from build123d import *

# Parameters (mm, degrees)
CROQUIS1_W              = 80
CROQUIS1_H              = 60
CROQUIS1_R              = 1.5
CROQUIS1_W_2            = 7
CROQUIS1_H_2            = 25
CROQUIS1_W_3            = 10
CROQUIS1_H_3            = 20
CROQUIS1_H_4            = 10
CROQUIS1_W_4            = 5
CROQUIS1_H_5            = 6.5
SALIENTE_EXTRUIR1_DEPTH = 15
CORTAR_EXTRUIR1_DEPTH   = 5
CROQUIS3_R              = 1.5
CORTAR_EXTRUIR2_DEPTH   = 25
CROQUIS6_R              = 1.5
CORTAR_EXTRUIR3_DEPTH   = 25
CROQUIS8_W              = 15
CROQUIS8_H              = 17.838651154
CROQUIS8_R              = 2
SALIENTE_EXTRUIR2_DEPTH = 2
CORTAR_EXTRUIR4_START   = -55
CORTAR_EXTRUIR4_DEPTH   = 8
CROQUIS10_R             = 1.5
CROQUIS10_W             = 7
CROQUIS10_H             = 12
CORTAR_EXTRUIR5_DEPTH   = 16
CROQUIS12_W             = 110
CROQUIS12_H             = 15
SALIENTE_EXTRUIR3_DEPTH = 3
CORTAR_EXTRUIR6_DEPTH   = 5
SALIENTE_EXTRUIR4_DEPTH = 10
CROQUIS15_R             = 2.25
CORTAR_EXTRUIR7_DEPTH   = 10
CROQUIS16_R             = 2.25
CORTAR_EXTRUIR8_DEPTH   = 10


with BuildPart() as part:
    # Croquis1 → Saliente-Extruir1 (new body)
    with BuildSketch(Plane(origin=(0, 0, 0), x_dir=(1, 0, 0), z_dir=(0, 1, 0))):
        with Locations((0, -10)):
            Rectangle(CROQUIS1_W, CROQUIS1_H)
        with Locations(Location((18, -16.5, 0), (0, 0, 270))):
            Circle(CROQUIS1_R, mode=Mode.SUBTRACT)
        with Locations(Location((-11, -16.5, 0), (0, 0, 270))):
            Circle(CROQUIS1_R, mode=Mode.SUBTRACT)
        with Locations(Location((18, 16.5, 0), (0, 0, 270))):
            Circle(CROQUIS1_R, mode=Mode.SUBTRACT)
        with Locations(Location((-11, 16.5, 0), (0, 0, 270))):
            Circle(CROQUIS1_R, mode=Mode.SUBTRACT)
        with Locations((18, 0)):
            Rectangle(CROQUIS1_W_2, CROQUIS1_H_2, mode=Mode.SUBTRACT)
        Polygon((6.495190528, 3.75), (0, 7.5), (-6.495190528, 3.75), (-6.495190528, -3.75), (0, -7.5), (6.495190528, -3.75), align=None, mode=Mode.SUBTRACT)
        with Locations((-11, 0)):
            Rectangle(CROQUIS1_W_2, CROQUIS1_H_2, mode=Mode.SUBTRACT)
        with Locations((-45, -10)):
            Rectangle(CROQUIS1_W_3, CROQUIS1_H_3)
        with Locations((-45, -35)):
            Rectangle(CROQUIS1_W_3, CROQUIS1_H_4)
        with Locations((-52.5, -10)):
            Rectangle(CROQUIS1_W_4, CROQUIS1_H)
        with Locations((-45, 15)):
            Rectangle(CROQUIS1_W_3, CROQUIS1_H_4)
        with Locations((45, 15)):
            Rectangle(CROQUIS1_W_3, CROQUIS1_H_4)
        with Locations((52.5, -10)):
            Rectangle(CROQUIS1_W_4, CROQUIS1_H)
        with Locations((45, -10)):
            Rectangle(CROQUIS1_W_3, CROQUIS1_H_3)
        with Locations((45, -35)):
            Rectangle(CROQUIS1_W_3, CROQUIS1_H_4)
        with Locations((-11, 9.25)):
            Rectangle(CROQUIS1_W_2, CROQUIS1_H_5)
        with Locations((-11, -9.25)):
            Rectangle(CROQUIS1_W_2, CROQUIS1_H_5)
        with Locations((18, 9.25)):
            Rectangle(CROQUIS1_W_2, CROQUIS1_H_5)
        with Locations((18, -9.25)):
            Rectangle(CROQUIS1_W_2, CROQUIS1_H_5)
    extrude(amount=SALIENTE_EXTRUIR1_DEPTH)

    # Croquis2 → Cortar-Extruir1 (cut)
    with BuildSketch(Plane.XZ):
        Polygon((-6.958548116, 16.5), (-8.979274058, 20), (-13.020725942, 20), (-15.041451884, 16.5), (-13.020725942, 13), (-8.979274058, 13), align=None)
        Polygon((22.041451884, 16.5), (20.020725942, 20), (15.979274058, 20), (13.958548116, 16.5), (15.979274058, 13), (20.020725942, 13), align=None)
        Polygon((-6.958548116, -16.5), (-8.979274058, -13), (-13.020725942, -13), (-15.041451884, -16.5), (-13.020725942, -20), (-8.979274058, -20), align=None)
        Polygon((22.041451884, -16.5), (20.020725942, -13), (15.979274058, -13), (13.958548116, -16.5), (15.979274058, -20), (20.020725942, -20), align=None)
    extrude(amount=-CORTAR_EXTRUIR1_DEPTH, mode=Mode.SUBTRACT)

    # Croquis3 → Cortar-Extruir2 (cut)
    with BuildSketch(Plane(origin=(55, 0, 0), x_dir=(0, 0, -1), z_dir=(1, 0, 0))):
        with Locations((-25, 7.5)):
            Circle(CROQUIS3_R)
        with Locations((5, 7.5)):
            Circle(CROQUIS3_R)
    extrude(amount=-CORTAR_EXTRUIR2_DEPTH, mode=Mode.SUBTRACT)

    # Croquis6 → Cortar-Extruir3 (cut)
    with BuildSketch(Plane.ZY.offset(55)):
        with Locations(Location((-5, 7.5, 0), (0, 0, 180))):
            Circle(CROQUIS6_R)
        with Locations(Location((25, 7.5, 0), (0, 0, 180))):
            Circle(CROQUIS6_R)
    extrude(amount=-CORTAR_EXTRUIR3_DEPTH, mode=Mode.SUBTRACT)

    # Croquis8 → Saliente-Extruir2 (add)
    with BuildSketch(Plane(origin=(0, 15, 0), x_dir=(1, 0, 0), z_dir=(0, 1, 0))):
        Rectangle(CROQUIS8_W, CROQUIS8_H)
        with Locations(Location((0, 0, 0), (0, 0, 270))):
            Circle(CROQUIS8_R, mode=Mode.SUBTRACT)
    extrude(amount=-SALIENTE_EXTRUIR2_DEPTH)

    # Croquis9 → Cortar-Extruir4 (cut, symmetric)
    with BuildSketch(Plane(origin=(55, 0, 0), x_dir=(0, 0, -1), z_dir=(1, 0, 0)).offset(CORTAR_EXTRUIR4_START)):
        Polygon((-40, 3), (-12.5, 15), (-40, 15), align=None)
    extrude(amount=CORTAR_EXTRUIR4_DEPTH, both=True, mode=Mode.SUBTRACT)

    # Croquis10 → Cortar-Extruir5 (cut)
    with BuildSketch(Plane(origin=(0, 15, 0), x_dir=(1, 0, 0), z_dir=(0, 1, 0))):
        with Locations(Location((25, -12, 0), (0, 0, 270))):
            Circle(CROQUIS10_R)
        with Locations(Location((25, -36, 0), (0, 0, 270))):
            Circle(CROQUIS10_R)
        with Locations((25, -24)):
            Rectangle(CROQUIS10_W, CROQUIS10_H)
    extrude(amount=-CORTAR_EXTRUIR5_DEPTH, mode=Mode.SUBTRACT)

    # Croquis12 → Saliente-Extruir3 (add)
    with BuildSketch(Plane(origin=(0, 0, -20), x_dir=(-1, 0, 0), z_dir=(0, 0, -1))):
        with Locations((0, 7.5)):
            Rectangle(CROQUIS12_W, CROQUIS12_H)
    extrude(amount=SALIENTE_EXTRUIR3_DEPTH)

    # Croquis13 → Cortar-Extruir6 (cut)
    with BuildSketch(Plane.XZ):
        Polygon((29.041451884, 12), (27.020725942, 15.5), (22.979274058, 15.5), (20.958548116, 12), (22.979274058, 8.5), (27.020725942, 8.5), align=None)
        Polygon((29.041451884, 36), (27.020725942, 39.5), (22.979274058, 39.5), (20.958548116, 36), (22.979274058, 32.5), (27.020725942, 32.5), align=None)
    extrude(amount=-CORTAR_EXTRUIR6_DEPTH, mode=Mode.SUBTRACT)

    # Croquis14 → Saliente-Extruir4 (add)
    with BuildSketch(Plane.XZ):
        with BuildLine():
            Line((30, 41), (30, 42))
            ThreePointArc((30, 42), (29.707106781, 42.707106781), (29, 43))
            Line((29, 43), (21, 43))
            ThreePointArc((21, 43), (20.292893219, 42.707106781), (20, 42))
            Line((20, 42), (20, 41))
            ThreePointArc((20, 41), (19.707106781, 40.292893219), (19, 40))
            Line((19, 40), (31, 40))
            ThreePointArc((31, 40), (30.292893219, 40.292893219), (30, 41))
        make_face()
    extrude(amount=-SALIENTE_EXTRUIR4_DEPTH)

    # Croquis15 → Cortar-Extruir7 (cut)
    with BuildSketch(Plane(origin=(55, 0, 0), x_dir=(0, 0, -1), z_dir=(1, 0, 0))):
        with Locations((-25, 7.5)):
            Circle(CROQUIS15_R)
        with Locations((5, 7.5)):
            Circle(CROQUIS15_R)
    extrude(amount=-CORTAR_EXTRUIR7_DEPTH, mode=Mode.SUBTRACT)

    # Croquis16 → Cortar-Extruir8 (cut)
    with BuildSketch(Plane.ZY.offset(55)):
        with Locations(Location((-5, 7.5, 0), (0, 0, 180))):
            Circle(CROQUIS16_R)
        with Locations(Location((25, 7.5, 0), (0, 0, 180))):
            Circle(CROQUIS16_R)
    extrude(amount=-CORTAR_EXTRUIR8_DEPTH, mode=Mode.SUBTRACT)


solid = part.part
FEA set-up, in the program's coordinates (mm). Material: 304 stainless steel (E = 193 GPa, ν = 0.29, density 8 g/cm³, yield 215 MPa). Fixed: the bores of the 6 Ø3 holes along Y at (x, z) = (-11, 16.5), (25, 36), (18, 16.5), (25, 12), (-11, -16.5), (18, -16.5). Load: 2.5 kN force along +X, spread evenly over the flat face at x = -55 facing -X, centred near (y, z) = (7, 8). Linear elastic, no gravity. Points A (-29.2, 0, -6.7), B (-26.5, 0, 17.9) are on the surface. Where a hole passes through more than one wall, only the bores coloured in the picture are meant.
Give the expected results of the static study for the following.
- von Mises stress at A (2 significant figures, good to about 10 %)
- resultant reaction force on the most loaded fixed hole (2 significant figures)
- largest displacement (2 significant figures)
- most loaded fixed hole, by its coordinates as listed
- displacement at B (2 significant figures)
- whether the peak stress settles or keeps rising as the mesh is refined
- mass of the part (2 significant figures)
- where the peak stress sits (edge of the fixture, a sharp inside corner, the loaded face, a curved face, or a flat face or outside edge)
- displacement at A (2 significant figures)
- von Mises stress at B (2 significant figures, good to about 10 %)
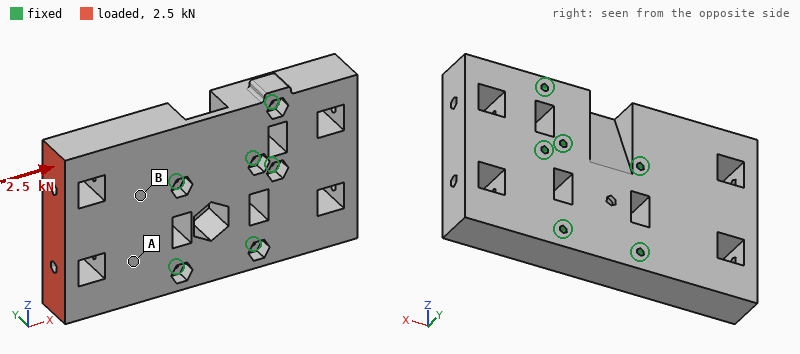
1.6 MPa
1.2 kN
1.8 µm
(-11, 16.5)
0.68 µm
keeps rising
700 g
edge of the fixture
0.63 µm
3.6 MPa
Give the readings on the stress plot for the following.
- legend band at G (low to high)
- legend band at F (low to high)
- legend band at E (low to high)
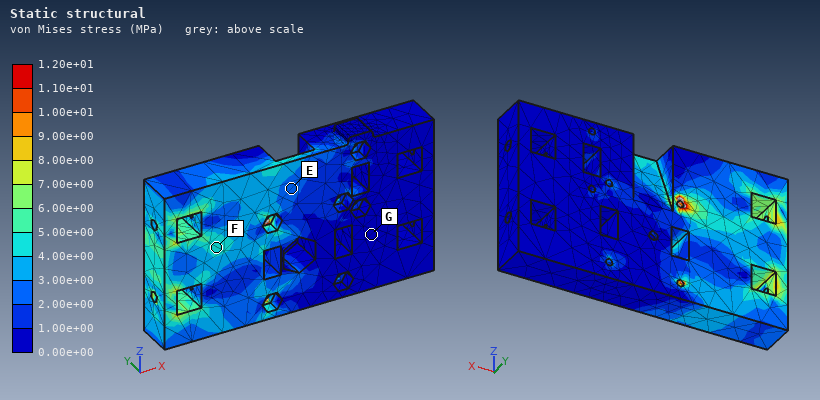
0.00e+00 to 1.00e+00 MPa
4.00e+00 to 5.00e+00 MPa
2.00e+00 to 3.00e+00 MPa
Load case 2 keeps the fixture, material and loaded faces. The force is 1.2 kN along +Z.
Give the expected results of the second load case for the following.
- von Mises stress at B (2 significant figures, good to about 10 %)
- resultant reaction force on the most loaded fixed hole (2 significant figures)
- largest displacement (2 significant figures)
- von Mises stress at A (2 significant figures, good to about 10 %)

3.7 MPa
1.3 kN
4.2 µm
5.8 MPa
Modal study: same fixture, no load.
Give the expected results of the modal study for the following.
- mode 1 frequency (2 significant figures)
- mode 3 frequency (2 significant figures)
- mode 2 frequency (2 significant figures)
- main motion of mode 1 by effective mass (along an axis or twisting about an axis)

4000 Hz
7000 Hz
6800 Hz
along Y
